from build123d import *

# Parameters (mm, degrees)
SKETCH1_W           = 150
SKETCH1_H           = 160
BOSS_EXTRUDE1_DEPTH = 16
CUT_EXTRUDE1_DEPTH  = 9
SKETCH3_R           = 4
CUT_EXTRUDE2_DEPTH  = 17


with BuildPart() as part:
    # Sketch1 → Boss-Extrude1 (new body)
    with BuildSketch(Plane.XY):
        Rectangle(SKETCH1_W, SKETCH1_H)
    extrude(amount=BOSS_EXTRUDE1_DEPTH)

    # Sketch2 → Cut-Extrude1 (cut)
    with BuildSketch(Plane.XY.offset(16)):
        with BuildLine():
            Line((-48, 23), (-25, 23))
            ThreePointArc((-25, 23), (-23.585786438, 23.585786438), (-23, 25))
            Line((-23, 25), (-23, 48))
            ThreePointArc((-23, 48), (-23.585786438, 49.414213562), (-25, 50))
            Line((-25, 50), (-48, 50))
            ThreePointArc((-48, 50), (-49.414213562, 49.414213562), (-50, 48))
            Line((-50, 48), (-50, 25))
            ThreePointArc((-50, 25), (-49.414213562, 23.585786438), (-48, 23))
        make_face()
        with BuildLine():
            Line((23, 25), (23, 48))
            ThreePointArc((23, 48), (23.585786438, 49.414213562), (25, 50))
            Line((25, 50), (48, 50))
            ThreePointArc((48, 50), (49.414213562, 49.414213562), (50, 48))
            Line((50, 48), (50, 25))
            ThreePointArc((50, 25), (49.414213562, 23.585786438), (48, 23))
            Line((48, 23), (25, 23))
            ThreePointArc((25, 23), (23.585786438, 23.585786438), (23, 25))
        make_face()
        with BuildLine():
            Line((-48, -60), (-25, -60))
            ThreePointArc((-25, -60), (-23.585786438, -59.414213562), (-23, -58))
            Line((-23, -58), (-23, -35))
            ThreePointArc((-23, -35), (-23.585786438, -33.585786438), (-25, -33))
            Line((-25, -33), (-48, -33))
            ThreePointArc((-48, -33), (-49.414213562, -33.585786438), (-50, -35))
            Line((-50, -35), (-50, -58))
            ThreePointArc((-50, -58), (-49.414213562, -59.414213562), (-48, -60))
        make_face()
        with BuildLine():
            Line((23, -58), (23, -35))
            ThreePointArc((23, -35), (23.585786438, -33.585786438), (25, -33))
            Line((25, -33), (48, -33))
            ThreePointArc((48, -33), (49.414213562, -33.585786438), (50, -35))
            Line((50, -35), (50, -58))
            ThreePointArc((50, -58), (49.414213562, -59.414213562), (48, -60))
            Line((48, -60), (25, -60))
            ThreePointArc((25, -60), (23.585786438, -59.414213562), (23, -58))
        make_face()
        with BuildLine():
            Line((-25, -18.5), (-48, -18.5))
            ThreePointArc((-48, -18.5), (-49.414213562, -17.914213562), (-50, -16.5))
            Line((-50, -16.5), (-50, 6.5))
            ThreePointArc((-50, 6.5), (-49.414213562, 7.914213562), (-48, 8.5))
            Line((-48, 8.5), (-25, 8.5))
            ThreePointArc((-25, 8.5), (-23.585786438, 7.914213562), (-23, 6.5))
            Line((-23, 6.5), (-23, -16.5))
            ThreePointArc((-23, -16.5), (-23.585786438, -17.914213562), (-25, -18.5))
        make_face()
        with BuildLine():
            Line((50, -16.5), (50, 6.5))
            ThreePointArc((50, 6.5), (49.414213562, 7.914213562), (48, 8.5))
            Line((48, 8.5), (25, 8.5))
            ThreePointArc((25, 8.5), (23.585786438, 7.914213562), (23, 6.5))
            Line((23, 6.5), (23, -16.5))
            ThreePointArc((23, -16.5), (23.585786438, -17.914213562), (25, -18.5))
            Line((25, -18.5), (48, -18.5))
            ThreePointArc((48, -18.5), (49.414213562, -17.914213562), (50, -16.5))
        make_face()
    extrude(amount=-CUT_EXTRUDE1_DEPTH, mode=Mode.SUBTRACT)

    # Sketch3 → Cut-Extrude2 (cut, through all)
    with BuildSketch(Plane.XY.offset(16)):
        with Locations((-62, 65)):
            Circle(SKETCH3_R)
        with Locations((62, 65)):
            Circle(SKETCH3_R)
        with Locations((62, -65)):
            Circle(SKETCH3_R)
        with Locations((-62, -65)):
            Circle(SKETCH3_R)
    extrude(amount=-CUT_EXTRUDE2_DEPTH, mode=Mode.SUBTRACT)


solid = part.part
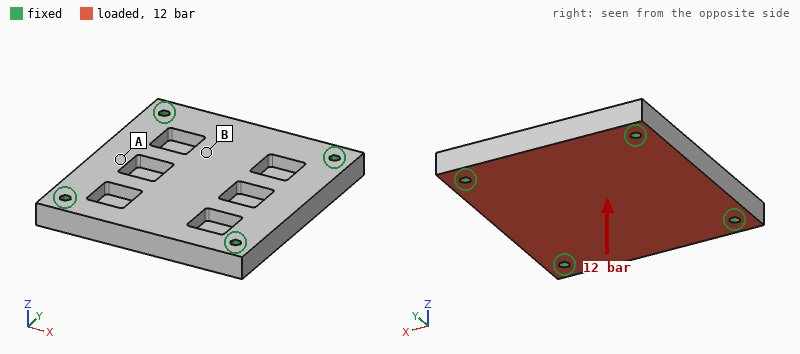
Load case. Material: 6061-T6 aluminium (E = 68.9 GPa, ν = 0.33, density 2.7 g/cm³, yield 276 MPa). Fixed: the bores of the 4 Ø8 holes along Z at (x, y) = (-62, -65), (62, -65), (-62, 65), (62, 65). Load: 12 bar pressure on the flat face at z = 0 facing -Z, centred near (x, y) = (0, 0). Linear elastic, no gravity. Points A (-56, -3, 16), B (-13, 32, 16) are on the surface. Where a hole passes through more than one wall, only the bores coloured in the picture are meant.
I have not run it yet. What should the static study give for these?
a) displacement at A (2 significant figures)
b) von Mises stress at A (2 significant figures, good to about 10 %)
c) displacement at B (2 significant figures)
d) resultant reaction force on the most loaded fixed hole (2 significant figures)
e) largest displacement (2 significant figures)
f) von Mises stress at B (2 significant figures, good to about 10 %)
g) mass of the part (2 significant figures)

0.088 mm
38 MPa
0.11 mm
7.3 kN
0.13 mm
20 MPa
920 g
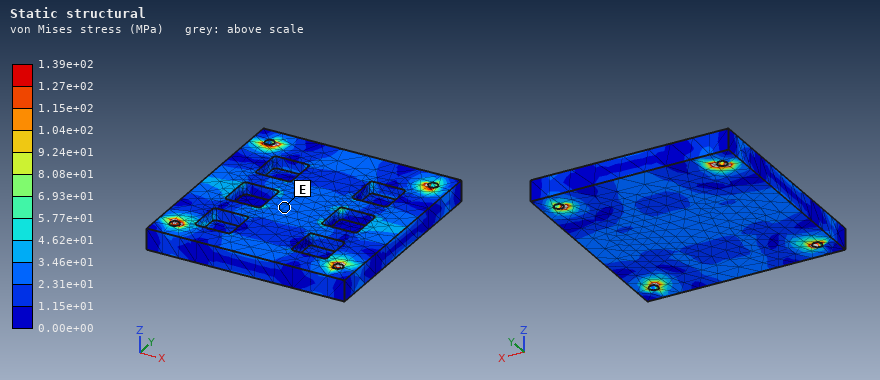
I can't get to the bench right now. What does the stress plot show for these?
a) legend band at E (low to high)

2.31e+01 to 3.46e+01 MPa
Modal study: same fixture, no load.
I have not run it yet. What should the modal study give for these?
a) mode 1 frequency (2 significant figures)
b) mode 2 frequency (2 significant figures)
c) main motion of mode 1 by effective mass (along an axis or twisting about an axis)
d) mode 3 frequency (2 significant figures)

2900 Hz
4700 Hz
along Z
4800 Hz
